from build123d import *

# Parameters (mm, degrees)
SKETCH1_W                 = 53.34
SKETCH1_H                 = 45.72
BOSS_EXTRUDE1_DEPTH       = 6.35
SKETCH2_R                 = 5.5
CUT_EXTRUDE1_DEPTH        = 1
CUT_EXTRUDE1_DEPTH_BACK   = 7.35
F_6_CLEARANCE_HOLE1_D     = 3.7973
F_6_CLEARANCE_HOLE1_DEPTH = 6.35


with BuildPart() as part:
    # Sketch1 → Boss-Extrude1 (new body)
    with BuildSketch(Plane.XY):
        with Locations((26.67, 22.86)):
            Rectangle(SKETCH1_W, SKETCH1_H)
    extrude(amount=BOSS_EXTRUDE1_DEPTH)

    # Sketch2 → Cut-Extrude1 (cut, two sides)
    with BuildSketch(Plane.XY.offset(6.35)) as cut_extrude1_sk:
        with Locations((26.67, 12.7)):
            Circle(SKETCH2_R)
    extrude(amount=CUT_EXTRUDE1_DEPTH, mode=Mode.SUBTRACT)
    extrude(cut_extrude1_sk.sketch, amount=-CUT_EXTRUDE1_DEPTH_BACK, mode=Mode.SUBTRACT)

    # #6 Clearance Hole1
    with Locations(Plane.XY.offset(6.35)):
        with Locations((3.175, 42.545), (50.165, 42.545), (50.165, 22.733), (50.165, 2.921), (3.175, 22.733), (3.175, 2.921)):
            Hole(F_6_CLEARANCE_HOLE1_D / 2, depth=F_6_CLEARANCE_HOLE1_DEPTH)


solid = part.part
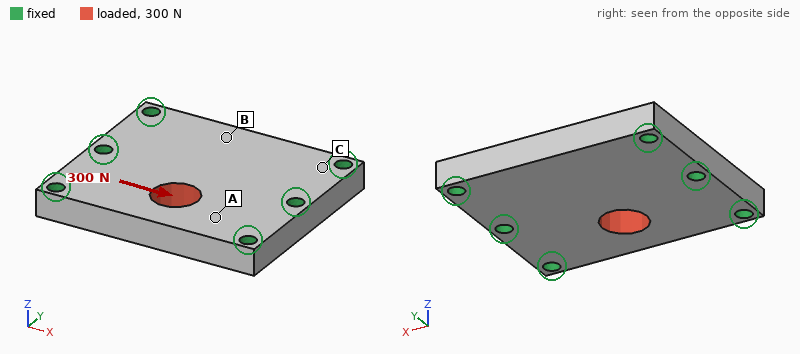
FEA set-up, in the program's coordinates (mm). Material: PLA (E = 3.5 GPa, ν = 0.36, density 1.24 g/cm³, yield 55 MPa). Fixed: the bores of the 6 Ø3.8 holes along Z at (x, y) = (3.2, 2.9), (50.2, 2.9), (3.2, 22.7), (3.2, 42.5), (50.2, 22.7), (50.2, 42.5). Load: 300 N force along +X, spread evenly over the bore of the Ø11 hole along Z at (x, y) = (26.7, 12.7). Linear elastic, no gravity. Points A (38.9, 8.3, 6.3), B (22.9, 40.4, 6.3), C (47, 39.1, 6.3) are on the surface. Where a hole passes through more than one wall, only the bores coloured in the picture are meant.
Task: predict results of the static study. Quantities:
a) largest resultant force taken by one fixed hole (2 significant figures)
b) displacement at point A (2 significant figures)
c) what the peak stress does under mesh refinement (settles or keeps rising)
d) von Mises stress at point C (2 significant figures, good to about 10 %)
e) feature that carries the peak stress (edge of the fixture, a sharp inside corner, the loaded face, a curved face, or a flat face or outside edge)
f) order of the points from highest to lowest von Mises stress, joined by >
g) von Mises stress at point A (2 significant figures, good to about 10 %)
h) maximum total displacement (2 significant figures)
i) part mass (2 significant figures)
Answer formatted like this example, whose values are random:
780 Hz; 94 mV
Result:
74 N; 4.0 µm; keeps rising; 0.42 MPa; edge of the fixture; A > C > B; 1.1 MPa; 7.5 µm; 18 g
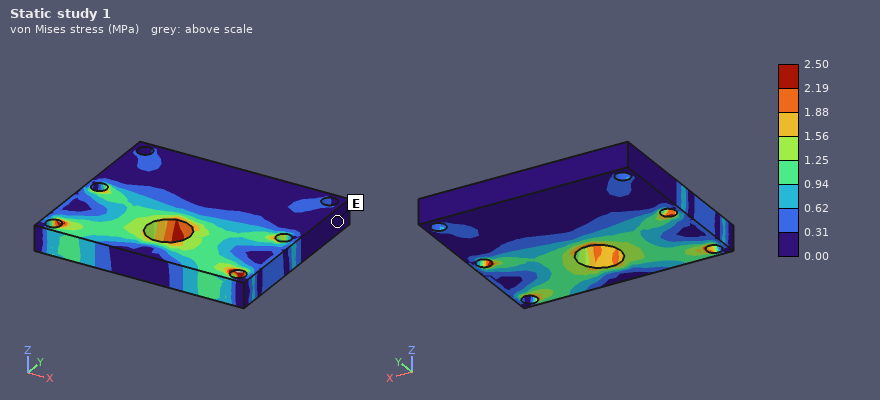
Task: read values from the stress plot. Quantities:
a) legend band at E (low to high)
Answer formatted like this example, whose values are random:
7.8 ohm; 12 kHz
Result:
0.00 to 0.31 MPa
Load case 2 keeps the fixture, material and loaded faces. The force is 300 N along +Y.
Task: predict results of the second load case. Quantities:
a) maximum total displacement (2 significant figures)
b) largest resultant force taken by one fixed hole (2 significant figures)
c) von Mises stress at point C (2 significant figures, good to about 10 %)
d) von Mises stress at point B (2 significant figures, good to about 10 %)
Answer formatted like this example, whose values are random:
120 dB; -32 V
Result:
17 µm; 76 N; 1.1 MPa; 0.32 MPa
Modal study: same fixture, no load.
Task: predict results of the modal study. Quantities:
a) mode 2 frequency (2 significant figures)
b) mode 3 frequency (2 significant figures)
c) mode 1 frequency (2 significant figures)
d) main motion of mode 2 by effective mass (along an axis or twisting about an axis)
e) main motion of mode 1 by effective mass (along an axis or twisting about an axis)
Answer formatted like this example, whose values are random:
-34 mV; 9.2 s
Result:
5300 Hz; 8400 Hz; 4300 Hz; twisting about X; along Z
